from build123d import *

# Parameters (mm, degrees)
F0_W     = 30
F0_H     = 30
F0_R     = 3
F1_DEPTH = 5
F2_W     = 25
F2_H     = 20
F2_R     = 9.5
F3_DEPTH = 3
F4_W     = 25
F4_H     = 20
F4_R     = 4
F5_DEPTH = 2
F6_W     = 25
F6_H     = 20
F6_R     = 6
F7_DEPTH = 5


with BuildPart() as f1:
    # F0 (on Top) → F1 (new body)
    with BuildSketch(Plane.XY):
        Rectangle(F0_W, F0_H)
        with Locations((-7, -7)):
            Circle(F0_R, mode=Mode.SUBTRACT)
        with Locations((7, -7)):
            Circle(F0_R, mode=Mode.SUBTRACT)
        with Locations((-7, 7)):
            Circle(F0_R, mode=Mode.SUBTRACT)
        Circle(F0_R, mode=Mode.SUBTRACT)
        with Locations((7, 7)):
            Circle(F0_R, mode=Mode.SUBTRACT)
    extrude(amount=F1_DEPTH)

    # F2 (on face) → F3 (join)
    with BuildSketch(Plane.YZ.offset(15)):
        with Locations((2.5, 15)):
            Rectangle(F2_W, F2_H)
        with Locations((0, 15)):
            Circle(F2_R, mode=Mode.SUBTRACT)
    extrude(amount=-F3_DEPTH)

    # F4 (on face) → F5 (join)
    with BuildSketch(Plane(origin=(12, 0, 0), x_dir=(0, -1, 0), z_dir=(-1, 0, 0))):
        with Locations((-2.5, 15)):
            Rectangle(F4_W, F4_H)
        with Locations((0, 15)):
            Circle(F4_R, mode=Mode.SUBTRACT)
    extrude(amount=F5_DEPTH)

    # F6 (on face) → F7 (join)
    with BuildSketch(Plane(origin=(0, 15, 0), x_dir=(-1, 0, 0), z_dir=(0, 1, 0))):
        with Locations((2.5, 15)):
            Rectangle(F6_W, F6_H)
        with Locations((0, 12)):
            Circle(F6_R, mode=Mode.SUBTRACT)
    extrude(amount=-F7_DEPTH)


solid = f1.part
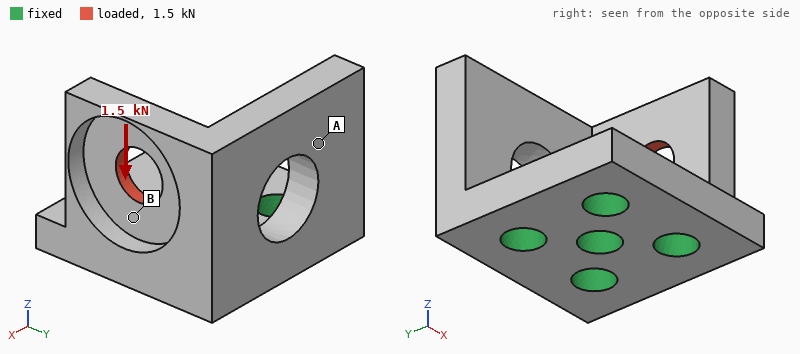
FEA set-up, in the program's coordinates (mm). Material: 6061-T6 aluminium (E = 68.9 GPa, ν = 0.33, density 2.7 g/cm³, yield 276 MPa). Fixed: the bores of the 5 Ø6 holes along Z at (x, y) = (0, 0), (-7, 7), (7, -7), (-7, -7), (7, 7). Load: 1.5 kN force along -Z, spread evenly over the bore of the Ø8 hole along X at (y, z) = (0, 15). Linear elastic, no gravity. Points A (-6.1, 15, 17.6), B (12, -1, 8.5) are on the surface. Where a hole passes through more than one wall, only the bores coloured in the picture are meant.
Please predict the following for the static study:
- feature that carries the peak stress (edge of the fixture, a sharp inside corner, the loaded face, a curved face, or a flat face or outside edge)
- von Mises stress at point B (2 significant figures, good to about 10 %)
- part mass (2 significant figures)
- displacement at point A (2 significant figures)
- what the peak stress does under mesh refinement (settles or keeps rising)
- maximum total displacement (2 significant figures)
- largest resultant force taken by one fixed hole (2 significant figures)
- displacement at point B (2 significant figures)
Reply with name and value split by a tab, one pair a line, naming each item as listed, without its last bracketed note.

feature that carries the peak stress	edge of the fixture
von Mises stress at point B	27 MPa
part mass	20 g
displacement at point A	2.1 µm
what the peak stress does under mesh refinement	keeps rising
maximum total displacement	13 µm
largest resultant force taken by one fixed hole	800 N
displacement at point B	3.5 µm
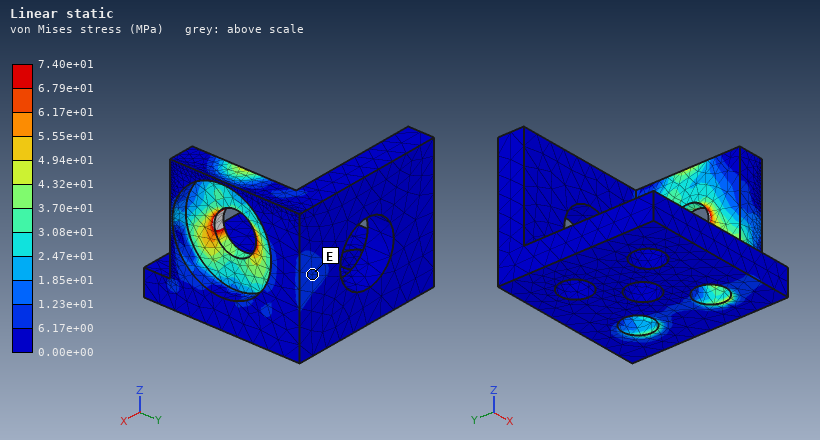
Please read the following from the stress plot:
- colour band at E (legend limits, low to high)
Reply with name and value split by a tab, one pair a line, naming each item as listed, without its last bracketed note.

colour band at E	6.17e+00 to 1.23e+01 MPa
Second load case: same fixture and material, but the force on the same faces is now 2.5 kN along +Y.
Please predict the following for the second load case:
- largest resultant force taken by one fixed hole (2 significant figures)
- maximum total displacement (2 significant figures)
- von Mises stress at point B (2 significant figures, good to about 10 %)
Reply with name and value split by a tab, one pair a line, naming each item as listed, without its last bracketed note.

largest resultant force taken by one fixed hole	2.0 kN
maximum total displacement	60 µm
von Mises stress at point B	140 MPa
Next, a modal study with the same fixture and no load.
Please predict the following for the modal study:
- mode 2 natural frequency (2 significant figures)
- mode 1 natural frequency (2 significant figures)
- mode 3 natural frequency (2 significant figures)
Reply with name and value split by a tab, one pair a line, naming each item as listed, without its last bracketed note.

mode 2 natural frequency	9900 Hz
mode 1 natural frequency	8600 Hz
mode 3 natural frequency	14 kHz
